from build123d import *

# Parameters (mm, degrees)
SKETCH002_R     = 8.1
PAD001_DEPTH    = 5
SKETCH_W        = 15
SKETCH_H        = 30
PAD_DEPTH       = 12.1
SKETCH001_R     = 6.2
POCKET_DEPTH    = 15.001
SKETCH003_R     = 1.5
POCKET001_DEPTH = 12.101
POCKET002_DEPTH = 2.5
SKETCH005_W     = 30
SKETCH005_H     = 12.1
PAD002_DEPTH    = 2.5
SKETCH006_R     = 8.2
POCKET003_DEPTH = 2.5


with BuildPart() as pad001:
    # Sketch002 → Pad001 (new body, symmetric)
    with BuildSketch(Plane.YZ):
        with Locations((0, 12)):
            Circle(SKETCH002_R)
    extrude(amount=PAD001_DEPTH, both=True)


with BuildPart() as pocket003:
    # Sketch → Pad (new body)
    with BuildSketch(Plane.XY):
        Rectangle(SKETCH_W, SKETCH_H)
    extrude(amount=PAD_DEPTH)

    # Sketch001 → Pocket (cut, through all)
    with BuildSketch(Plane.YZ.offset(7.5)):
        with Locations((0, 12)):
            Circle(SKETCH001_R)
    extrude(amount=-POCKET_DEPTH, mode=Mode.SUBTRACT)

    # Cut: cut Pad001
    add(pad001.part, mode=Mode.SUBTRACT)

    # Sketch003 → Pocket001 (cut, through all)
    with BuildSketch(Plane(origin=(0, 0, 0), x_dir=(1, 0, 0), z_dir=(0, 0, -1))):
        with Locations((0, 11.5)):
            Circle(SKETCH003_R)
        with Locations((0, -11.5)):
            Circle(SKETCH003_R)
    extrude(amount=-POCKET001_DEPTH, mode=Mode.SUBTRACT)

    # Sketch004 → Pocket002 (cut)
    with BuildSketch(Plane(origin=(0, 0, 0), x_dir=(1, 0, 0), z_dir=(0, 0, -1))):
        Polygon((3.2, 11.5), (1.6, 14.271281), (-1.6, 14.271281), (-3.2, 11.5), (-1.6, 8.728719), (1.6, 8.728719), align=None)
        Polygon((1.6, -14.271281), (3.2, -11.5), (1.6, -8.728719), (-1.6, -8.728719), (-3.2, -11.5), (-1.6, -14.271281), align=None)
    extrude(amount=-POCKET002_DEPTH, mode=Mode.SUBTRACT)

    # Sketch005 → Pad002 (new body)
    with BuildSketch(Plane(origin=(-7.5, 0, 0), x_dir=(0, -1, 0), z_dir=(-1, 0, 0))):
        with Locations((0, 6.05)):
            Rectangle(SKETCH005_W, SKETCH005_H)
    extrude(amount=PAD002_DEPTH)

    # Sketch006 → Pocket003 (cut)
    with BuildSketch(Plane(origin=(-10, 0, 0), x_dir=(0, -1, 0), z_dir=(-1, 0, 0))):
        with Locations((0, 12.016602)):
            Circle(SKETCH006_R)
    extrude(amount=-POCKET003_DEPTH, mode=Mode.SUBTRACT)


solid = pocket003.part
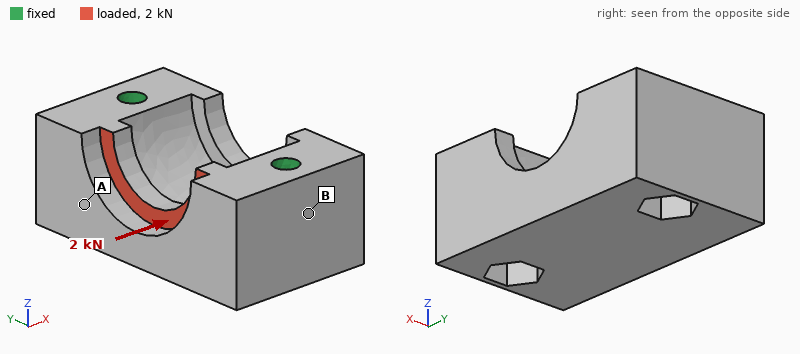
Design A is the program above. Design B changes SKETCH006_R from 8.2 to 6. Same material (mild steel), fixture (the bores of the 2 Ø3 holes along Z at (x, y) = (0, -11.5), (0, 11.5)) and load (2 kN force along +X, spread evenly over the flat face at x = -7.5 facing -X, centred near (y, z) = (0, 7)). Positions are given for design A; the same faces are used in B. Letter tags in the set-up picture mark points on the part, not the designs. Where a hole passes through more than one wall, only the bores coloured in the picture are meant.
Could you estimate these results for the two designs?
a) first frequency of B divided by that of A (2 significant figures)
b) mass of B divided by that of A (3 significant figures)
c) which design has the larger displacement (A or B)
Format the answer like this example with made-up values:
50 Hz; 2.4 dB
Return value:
0.98; 1.03; B
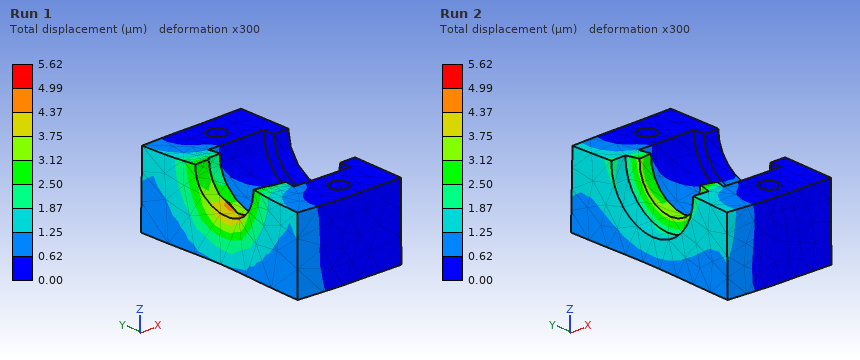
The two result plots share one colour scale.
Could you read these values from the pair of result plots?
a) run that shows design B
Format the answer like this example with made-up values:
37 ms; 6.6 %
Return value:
Run 1
